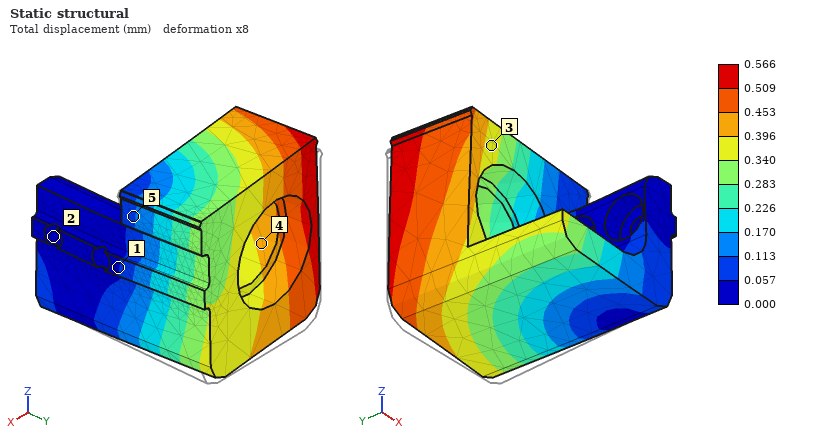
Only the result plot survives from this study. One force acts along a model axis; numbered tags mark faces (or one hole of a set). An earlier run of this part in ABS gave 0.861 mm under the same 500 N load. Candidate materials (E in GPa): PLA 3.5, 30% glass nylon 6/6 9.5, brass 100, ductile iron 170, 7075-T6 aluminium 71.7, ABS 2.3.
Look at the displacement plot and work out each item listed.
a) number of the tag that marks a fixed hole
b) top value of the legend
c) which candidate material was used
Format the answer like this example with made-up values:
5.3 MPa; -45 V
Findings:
2; 0.566 mm; PLA
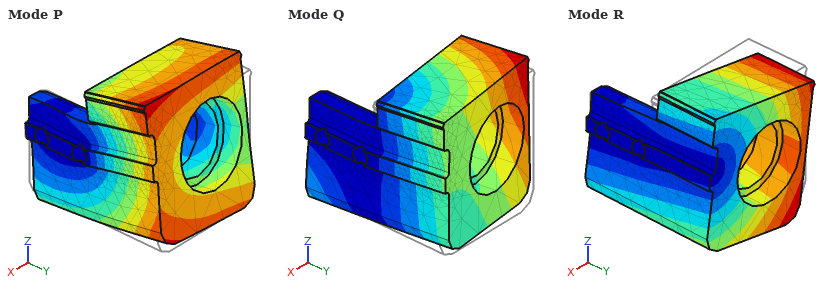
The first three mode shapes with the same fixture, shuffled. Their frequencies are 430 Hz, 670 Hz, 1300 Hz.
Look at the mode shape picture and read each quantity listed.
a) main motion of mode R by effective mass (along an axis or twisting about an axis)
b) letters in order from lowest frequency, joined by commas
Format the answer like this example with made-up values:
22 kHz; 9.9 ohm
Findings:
along Z; R, Q, P
